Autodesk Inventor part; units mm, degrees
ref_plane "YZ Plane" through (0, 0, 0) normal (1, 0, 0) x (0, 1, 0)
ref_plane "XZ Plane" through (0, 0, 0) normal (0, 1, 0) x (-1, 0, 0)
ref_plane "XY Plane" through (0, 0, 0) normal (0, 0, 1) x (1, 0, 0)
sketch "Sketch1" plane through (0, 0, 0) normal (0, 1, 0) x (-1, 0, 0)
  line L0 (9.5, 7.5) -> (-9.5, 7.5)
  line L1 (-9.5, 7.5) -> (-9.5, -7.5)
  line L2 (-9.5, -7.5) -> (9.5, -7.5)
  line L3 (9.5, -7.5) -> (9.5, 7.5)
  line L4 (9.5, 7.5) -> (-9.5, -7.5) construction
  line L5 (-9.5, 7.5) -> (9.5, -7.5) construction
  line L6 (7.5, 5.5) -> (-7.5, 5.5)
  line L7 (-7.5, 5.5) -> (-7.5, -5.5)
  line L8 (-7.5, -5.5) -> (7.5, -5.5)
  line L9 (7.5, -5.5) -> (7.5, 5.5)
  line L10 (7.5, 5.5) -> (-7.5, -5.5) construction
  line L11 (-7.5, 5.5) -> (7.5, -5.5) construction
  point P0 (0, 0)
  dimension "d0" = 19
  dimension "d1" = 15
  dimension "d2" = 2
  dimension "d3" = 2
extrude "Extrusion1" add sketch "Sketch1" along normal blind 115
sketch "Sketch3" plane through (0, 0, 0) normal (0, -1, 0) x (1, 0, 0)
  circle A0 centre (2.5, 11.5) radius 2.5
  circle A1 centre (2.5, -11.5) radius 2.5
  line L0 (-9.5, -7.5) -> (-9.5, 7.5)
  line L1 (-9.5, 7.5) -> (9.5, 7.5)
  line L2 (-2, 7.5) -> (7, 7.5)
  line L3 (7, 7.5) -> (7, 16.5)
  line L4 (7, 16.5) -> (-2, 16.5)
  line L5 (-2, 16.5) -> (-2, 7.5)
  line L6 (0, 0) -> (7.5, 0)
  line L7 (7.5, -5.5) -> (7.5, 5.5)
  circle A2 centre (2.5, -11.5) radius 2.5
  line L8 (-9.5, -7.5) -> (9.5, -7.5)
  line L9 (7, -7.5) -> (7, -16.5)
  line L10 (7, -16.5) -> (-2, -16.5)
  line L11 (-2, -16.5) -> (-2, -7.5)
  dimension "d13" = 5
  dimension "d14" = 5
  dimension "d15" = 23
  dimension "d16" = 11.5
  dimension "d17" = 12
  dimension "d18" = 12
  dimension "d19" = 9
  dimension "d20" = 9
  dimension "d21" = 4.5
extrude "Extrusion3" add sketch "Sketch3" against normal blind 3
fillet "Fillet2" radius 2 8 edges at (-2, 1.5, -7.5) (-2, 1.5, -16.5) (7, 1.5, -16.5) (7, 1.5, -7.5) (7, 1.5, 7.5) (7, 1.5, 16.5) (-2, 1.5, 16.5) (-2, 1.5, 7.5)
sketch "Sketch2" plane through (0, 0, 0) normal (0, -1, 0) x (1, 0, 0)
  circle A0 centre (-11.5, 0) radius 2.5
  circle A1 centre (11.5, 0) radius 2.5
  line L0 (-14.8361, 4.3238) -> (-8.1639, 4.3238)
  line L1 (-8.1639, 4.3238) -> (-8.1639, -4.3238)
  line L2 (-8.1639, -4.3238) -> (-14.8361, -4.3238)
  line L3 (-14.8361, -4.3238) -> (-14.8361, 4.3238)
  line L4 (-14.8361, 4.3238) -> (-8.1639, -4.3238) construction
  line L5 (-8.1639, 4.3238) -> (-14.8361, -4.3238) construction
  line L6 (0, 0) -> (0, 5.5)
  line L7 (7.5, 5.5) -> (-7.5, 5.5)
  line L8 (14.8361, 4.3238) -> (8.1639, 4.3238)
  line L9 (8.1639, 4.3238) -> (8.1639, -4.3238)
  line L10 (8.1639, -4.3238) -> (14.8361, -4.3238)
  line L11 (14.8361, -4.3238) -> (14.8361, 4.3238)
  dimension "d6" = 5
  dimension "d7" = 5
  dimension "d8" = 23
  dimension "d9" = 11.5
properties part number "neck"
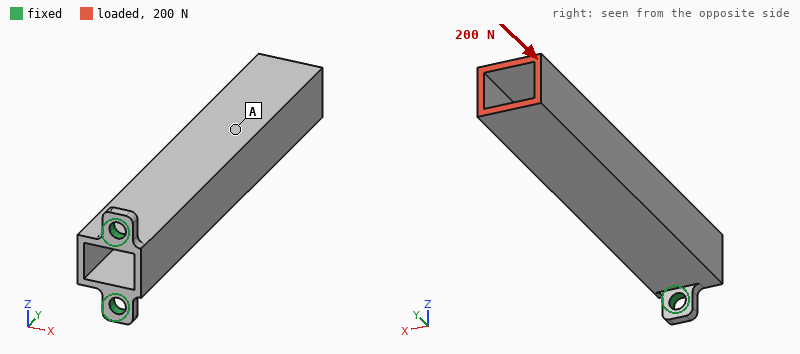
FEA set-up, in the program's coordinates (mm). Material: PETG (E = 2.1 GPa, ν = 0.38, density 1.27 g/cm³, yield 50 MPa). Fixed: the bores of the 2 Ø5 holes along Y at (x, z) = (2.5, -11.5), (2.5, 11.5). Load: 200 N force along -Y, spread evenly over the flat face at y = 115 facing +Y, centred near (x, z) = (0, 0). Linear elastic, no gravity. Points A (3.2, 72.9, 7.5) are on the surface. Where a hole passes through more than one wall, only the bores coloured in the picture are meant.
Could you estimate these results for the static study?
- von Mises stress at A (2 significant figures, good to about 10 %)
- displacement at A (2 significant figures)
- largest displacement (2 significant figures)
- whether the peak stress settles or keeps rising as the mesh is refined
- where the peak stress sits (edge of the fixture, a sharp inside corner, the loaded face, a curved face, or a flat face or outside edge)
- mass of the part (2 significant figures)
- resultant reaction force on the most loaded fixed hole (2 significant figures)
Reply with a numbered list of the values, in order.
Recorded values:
1. 1.7 MPa
2. 0.76 mm
3. 1.2 mm
4. keeps rising
5. edge of the fixture
6. 18 g
7. 100 N
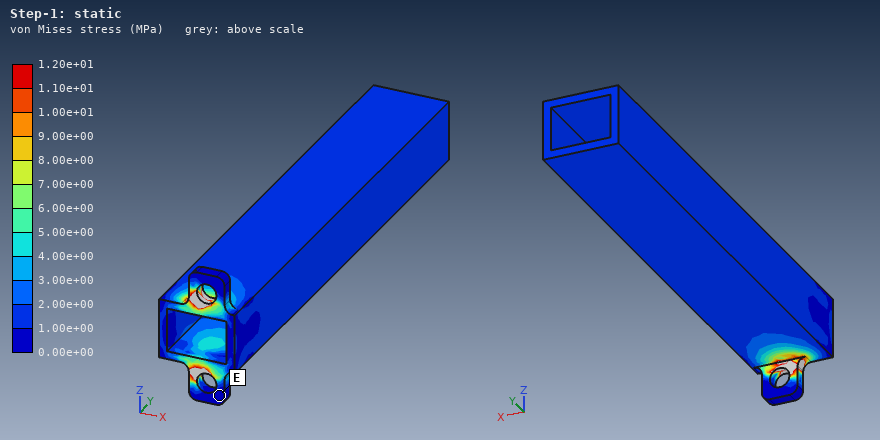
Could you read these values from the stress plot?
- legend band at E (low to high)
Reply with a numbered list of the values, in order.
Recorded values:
1. 0.00e+00 to 1.00e+00 MPa
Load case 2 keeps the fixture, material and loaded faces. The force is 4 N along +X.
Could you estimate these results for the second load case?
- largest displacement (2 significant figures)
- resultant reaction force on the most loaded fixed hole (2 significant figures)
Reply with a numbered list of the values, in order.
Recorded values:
1. 1.2 mm
2. 2.5 N
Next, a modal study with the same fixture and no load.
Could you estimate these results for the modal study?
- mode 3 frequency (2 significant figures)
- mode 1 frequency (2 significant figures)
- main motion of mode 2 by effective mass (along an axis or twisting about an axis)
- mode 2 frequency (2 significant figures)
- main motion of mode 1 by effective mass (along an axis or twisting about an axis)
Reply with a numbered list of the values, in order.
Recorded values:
1. 1300 Hz
2. 120 Hz
3. along Z
4. 220 Hz
5. along X
